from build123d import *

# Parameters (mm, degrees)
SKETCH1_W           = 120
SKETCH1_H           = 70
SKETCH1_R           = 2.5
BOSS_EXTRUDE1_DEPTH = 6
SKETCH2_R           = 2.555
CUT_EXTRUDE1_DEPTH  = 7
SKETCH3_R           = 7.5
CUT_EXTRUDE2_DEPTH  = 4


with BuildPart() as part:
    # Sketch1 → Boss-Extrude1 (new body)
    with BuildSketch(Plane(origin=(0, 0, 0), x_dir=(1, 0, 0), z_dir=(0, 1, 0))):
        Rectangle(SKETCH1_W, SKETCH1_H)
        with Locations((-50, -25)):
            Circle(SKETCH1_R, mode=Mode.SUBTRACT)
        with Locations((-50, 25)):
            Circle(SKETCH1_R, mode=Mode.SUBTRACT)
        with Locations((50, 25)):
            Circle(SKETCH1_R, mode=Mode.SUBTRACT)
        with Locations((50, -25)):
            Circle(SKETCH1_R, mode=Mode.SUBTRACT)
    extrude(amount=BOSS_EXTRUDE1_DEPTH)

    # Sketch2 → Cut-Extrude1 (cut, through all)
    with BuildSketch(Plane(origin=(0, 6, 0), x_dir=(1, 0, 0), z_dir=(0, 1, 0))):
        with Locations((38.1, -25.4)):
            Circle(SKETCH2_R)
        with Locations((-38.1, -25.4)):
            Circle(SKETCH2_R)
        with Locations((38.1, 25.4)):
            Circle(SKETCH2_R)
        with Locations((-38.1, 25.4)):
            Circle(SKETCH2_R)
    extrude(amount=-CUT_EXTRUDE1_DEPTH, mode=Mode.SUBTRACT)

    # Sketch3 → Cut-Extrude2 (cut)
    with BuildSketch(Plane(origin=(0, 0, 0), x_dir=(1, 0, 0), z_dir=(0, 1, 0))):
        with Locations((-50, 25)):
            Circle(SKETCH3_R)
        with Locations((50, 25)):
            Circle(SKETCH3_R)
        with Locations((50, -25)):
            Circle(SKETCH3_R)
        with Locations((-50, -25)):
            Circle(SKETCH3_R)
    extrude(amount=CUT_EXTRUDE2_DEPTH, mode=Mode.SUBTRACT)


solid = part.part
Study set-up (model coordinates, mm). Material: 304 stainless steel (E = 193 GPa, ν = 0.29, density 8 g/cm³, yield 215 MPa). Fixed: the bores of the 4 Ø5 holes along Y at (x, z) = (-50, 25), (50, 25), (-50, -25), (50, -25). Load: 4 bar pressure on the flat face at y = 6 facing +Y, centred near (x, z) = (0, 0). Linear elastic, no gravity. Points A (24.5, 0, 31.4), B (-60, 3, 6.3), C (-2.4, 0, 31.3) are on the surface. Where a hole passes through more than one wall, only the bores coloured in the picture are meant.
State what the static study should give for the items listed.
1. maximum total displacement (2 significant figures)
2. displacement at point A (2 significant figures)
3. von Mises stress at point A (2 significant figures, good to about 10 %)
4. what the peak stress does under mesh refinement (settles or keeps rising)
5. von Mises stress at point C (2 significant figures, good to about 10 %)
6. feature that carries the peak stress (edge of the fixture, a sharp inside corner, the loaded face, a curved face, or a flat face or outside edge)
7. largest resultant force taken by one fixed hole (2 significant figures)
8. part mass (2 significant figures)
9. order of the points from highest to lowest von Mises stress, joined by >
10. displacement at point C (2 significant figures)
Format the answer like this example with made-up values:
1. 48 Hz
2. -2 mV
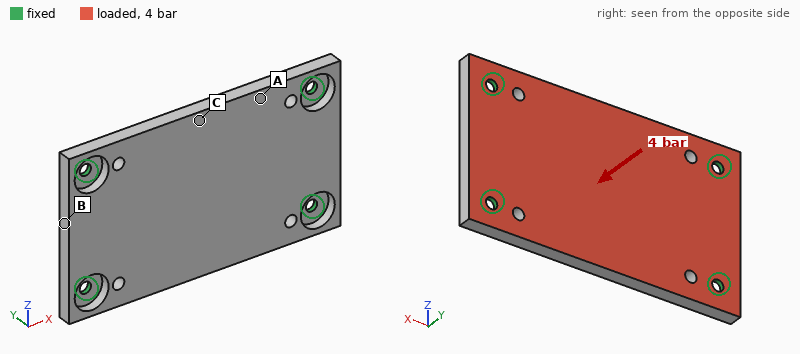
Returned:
1. 73 µm
2. 50 µm
3. 37 MPa
4. keeps rising
5. 54 MPa
6. edge of the fixture
7. 1.7 kN
8. 380 g
9. C > A > B
10. 72 µm
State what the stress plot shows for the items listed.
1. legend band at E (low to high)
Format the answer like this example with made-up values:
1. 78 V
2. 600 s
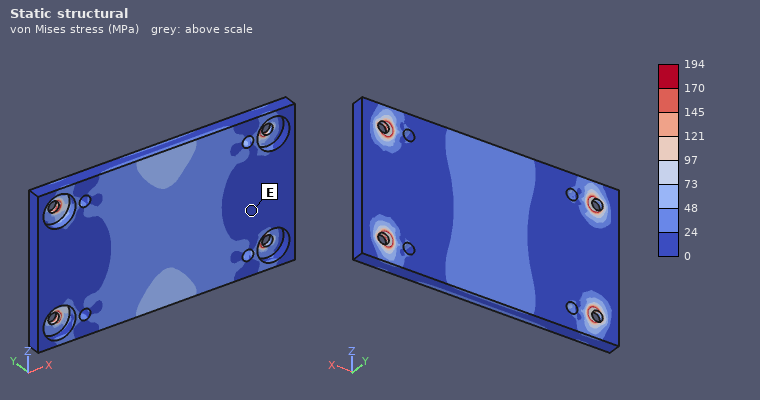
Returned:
1. 0 to 24 MPa
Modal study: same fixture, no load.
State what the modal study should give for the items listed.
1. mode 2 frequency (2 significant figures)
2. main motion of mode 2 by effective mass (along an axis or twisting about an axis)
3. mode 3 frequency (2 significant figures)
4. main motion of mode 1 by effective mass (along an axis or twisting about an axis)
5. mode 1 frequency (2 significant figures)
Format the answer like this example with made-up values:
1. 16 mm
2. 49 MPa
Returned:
1. 3100 Hz
2. twisting about X
3. 5300 Hz
4. along Y
5. 1900 Hz
